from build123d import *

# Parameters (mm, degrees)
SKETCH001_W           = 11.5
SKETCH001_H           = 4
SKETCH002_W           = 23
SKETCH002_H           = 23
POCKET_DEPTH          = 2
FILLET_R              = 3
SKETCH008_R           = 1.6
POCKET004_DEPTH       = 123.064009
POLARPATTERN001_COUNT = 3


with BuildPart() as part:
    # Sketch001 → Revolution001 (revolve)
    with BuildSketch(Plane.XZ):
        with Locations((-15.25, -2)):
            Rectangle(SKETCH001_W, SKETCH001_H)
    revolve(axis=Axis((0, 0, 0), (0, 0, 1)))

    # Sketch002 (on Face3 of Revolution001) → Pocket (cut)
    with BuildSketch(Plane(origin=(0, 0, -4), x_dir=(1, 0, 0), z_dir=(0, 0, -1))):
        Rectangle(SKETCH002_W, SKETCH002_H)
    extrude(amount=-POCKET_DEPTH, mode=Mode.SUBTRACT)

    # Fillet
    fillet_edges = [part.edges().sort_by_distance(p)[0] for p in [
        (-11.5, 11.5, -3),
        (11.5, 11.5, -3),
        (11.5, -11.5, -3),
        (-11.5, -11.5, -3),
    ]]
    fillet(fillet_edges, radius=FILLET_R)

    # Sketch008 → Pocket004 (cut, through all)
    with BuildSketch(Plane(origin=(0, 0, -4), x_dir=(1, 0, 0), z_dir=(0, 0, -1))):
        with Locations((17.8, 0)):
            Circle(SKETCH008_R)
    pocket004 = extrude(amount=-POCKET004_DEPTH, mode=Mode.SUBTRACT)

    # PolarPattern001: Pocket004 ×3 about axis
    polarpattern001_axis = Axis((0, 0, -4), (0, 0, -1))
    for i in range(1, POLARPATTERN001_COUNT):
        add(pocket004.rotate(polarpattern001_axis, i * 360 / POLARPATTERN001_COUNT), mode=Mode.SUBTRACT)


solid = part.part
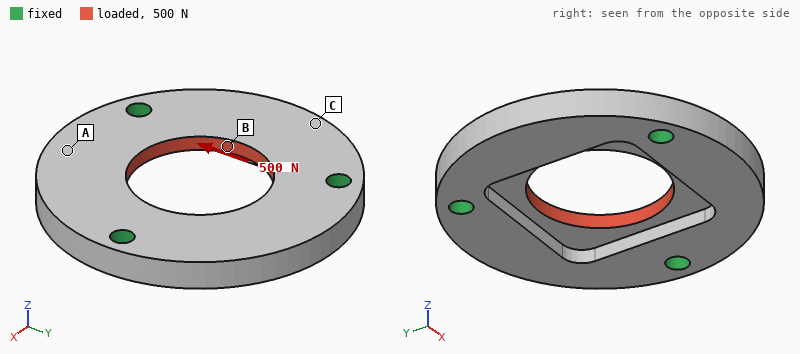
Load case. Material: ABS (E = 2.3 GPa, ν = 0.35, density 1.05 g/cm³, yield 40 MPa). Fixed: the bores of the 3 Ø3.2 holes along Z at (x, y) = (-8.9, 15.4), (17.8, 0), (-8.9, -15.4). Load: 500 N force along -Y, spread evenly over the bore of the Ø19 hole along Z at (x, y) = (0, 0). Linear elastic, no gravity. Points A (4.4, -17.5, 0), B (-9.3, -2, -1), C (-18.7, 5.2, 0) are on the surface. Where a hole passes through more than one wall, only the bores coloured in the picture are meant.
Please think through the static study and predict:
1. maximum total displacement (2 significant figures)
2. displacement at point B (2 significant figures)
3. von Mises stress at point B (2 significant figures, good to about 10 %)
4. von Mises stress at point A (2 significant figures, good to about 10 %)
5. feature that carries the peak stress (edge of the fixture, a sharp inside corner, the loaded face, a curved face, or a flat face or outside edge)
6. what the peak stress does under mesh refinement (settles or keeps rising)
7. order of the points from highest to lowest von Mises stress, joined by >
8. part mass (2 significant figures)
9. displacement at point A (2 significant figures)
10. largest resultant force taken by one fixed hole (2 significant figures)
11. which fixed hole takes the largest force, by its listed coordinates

58 µm
25 µm
7.2 MPa
3.0 MPa
edge of the fixture
keeps rising
B > A > C
4.0 g
47 µm
200 N
(17.8, 0)
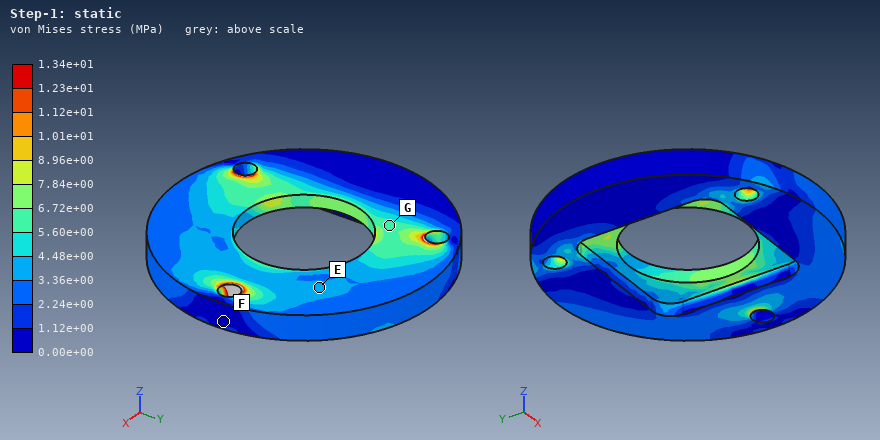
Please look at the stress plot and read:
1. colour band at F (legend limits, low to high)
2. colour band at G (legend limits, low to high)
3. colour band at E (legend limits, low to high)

0.00e+00 to 1.12e+00 MPa
5.60e+00 to 6.72e+00 MPa
3.36e+00 to 4.48e+00 MPa
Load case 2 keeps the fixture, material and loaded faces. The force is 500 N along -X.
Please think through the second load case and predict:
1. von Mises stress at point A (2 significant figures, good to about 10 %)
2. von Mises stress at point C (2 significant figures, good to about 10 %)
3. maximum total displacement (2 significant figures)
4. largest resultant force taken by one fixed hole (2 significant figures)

1.7 MPa
3.6 MPa
69 µm
190 N
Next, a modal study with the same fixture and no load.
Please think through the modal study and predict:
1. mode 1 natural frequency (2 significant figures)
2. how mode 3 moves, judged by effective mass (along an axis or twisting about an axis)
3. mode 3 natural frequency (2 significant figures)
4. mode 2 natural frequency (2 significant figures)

4000 Hz
along Z
4300 Hz
4100 Hz
